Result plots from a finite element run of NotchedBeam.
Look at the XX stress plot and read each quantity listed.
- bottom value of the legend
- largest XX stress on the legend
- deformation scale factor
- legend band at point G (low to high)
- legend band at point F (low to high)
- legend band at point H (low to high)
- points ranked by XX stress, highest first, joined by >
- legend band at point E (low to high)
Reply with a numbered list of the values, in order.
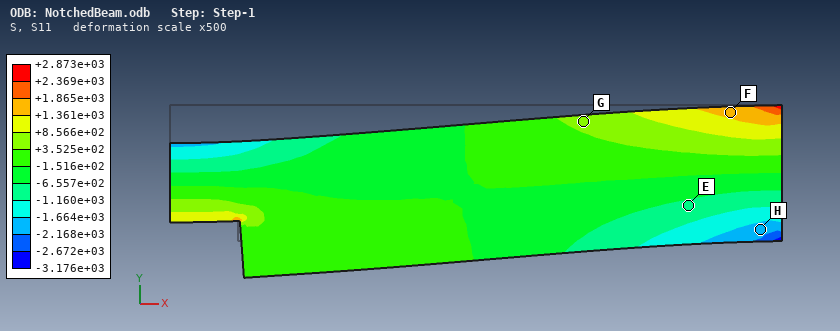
1. -3.176e+03
2. +2.873e+03
3. 500
4. +3.525e+02 to +8.566e+02
5. +1.361e+03 to +1.865e+03
6. -2.168e+03 to -1.664e+03
7. F > G > E > H
8. -1.160e+03 to -6.557e+02
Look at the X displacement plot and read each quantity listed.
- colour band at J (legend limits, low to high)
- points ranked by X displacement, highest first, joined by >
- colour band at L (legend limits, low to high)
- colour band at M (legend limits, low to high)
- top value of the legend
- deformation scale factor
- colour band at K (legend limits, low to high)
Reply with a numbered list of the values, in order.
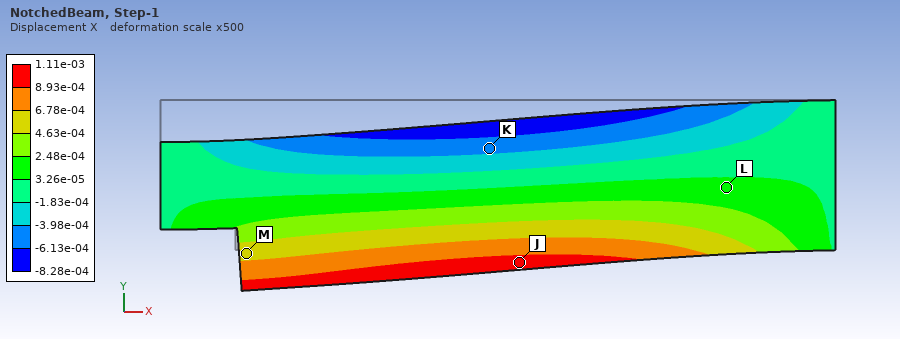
1. 8.93e-04 to 1.11e-03
2. J > M > L > K
3. 3.26e-05 to 2.48e-04
4. 4.63e-04 to 6.78e-04
5. 1.11e-03
6. 500
7. -6.13e-04 to -3.98e-04
